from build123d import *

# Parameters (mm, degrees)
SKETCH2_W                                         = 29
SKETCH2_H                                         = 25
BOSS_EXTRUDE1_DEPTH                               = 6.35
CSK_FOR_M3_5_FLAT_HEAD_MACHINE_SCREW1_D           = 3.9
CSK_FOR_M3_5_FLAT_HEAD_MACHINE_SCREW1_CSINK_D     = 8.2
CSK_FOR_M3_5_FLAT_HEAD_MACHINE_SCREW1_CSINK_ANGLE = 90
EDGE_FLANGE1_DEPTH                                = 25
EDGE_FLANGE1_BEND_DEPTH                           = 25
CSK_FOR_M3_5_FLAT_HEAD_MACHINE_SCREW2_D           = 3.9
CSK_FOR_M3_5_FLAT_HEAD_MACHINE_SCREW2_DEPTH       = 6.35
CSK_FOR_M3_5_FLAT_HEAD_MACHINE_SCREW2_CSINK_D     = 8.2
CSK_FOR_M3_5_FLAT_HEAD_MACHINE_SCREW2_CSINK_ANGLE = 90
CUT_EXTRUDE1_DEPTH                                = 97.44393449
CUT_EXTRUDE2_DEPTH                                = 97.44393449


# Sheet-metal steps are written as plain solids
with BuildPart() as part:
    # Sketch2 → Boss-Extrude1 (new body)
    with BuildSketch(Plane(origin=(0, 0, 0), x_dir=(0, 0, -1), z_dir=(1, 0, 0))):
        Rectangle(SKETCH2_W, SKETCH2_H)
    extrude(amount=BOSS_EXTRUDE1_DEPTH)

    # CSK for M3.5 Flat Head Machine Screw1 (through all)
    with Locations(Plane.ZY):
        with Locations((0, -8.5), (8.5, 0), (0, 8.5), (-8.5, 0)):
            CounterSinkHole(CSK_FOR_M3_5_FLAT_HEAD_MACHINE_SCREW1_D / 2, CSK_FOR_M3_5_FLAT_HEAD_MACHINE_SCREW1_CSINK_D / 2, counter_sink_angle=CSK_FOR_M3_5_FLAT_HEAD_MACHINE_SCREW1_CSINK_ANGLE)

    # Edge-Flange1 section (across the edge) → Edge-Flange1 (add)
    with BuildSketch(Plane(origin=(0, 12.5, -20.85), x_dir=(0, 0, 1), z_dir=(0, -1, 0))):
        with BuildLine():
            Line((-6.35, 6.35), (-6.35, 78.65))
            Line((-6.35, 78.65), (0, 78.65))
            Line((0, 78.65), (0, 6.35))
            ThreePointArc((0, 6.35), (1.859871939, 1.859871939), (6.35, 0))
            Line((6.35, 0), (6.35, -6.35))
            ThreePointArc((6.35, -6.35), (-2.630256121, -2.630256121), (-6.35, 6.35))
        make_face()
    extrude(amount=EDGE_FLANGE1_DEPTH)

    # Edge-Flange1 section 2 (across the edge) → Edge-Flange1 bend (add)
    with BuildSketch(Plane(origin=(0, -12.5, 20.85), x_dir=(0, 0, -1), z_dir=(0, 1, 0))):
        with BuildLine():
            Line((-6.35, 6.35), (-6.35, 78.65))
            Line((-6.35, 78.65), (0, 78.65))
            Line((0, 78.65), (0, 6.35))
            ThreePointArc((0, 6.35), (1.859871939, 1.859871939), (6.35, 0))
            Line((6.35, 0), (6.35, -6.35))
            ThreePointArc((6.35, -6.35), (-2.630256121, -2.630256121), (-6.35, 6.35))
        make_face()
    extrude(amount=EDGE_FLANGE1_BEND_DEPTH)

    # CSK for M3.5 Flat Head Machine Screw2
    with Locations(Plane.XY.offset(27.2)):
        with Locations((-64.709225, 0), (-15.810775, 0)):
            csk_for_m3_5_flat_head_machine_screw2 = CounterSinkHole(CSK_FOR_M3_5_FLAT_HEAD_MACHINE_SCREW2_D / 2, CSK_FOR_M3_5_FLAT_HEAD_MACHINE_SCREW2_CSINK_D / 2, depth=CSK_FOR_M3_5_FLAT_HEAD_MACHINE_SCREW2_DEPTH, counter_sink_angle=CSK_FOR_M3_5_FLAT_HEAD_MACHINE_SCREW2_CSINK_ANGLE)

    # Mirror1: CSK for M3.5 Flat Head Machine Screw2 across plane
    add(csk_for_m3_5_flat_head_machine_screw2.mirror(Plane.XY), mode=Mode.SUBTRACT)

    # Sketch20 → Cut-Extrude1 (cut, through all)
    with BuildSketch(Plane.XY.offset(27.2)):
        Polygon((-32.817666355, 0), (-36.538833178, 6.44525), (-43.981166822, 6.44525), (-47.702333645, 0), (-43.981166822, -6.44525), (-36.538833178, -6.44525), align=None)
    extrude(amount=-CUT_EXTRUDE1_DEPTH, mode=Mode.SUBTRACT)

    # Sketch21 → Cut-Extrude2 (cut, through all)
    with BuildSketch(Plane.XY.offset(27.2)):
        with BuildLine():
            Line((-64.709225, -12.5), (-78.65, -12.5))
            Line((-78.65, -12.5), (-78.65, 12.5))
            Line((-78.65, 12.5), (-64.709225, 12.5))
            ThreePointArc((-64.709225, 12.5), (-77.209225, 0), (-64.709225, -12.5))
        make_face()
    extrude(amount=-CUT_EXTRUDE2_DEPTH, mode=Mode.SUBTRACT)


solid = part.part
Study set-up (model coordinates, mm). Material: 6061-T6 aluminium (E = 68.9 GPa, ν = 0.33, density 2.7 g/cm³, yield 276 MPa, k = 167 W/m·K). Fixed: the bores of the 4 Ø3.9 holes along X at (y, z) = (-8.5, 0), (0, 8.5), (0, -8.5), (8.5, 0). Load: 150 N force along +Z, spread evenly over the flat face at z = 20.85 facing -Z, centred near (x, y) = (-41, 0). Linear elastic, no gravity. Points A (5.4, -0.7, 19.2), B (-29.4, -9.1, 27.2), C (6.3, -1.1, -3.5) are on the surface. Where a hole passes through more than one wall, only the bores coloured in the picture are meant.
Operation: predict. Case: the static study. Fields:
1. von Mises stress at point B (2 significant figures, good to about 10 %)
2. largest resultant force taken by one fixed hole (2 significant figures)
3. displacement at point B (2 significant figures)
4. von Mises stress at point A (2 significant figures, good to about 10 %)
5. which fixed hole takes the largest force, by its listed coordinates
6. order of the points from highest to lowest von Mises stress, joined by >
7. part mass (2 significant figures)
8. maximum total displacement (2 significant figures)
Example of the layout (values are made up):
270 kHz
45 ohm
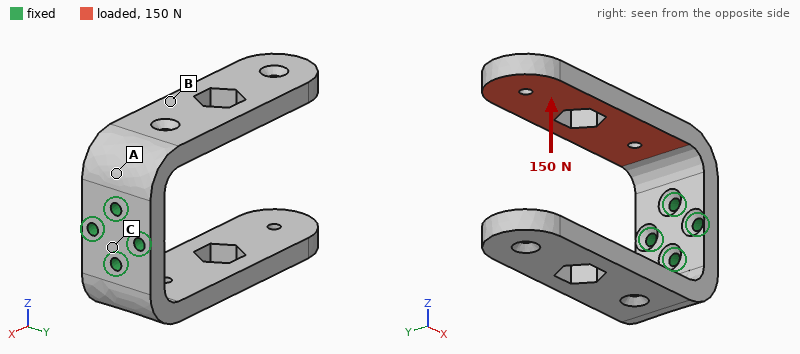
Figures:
17 MPa
430 N
0.16 mm
27 MPa
(0, 8.5)
A > B > C
76 g
0.52 mm
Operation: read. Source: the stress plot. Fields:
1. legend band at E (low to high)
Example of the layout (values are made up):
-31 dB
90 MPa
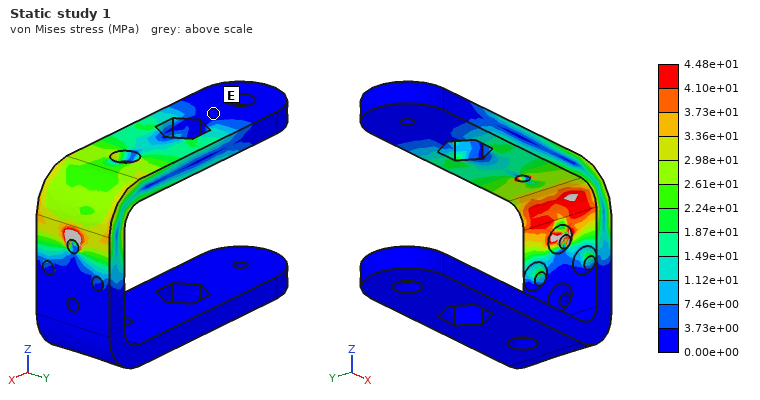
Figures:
0.00e+00 to 3.73e+00 MPa
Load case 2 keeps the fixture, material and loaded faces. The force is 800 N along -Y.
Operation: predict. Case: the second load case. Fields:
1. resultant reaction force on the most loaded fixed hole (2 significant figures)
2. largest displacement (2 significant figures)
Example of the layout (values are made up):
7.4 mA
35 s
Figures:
1.4 kN
0.97 mm
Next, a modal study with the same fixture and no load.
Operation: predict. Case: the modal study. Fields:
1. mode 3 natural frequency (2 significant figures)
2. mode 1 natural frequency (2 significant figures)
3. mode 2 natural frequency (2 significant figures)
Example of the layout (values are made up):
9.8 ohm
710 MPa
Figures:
1100 Hz
660 Hz
660 Hz
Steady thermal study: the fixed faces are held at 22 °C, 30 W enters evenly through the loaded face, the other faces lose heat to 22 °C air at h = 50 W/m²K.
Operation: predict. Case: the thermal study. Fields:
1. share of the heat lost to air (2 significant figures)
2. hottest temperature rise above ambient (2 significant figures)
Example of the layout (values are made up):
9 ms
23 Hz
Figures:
24 %
57 K
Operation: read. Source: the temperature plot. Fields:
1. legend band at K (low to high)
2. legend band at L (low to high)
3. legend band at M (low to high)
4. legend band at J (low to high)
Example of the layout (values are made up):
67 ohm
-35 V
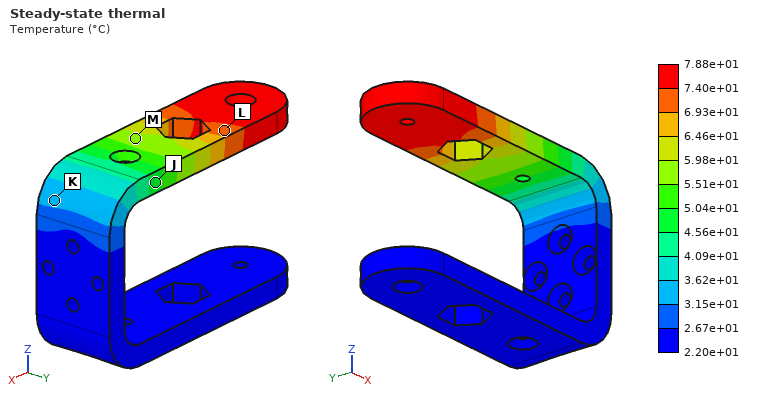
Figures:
3.15e+01 to 3.62e+01 °C
6.93e+01 to 7.40e+01 °C
5.51e+01 to 5.98e+01 °C
4.56e+01 to 5.04e+01 °C
